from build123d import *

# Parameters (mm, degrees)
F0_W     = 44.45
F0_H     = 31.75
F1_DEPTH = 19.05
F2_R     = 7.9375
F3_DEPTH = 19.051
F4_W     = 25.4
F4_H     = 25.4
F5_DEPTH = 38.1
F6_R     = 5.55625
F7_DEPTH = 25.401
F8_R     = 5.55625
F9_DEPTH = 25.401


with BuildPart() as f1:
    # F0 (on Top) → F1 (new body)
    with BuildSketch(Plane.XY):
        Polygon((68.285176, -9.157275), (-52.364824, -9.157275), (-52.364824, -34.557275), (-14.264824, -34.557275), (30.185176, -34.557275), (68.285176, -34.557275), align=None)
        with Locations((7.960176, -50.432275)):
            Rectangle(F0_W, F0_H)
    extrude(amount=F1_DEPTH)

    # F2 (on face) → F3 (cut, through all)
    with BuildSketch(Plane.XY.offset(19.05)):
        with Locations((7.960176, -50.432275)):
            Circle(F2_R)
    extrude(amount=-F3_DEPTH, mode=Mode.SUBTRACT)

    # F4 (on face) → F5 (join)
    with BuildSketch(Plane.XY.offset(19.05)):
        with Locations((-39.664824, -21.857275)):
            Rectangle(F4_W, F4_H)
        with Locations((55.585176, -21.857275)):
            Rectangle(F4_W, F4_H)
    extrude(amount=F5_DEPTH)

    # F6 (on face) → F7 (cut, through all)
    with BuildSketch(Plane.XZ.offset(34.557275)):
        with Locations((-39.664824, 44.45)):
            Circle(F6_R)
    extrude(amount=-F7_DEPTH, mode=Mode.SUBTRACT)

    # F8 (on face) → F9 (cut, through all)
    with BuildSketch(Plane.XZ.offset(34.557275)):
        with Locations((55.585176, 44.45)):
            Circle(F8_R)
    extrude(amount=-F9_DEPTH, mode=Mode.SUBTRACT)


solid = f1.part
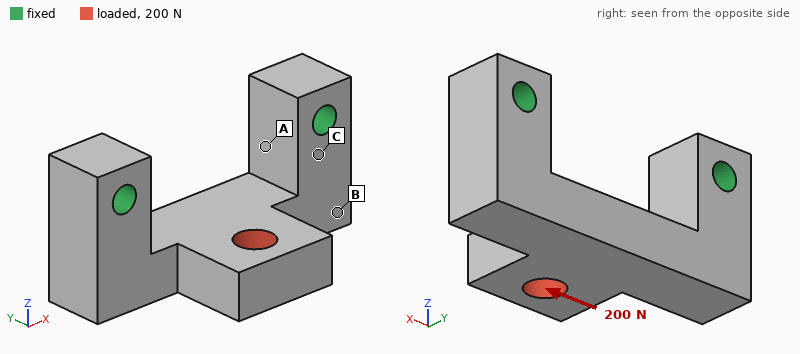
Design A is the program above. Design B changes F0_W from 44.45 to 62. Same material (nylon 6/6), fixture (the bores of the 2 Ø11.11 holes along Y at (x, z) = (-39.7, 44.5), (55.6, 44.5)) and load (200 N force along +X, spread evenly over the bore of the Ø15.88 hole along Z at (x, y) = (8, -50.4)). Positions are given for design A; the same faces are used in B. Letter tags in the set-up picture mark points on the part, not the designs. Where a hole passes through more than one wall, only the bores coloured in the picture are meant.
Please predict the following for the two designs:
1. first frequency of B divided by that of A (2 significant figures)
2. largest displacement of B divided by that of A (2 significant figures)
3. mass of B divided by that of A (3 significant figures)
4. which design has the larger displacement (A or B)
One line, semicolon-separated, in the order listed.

0.95; 0.74; 1.08; A
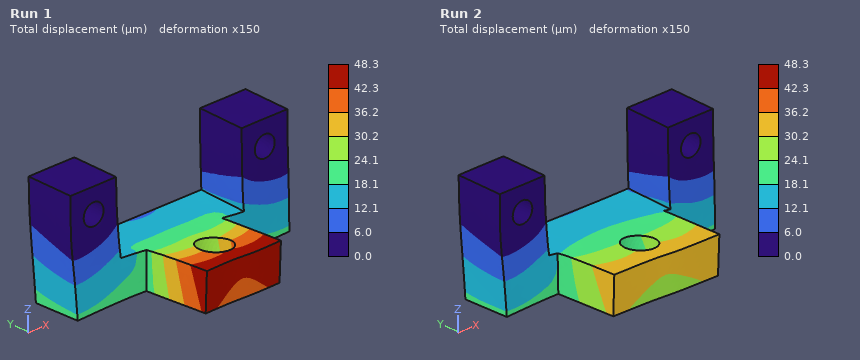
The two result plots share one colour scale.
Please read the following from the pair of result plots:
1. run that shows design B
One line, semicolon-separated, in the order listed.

Run 2
